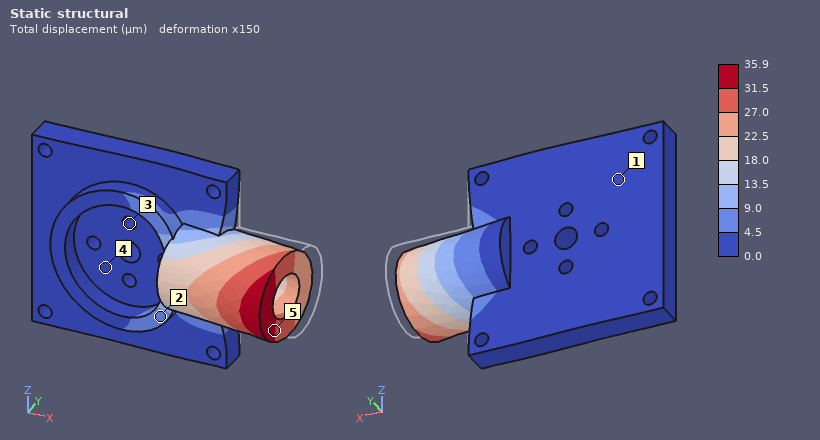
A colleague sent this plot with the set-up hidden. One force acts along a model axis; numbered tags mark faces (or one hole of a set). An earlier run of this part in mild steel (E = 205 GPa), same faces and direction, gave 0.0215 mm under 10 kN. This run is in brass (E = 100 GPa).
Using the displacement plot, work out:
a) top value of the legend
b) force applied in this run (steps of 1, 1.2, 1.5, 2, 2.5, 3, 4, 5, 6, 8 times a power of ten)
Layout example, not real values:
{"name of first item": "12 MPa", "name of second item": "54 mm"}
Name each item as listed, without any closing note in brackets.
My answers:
{"top value of the legend": "35.9 µm", "force applied in this run": "8 kN"}
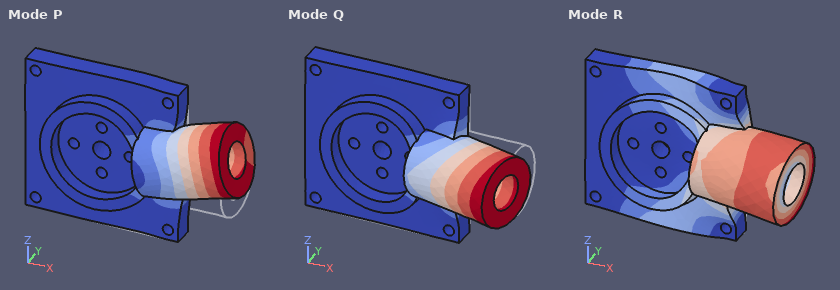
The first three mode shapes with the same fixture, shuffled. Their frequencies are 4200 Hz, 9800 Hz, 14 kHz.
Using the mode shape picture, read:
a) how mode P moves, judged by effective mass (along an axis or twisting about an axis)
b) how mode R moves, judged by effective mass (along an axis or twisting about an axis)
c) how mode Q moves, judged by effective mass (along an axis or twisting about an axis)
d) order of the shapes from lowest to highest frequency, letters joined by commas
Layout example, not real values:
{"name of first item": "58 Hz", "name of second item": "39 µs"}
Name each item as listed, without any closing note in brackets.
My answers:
{"how mode P moves, judged by effective mass": "along Z", "how mode R moves, judged by effective mass": "twisting about X", "how mode Q moves, judged by effective mass": "along Y", "order of the shapes from lowest to highest frequency, letters joined by commas": "Q, P, R"}
